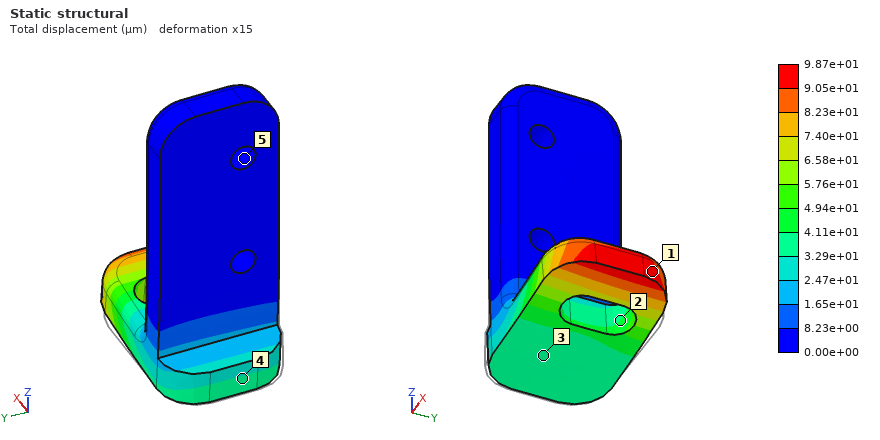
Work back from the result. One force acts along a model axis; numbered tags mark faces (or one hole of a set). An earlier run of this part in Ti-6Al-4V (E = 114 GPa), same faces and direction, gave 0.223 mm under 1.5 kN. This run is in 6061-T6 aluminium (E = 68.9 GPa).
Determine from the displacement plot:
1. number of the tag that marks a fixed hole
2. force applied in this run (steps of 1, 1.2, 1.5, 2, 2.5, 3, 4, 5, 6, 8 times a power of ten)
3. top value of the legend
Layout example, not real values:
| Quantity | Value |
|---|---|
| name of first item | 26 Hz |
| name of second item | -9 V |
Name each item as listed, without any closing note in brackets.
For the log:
| Quantity | Value |
|---|---|
| number of the tag that marks a fixed hole | 5 |
| force applied in this run | 400 N |
| top value of the legend | 9.87e+01 µm |
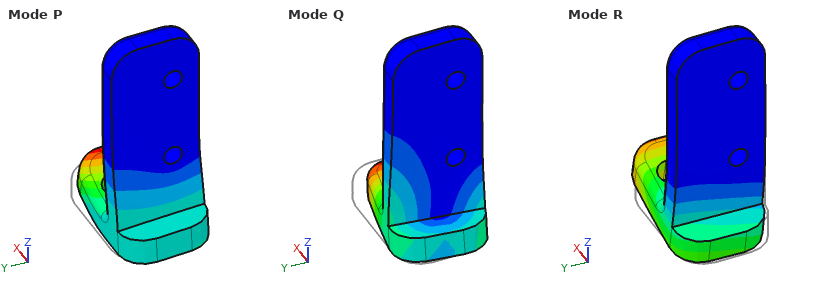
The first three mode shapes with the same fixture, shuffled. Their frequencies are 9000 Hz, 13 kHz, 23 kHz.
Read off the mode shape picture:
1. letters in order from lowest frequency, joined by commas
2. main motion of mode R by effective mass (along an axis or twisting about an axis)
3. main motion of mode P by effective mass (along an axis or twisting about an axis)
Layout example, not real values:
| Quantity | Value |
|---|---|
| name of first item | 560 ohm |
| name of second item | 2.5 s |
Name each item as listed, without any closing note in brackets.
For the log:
| Quantity | Value |
|---|---|
| letters in order from lowest frequency, joined by commas | R, Q, P |
| main motion of mode R by effective mass | along X |
| main motion of mode P by effective mass | along X |
